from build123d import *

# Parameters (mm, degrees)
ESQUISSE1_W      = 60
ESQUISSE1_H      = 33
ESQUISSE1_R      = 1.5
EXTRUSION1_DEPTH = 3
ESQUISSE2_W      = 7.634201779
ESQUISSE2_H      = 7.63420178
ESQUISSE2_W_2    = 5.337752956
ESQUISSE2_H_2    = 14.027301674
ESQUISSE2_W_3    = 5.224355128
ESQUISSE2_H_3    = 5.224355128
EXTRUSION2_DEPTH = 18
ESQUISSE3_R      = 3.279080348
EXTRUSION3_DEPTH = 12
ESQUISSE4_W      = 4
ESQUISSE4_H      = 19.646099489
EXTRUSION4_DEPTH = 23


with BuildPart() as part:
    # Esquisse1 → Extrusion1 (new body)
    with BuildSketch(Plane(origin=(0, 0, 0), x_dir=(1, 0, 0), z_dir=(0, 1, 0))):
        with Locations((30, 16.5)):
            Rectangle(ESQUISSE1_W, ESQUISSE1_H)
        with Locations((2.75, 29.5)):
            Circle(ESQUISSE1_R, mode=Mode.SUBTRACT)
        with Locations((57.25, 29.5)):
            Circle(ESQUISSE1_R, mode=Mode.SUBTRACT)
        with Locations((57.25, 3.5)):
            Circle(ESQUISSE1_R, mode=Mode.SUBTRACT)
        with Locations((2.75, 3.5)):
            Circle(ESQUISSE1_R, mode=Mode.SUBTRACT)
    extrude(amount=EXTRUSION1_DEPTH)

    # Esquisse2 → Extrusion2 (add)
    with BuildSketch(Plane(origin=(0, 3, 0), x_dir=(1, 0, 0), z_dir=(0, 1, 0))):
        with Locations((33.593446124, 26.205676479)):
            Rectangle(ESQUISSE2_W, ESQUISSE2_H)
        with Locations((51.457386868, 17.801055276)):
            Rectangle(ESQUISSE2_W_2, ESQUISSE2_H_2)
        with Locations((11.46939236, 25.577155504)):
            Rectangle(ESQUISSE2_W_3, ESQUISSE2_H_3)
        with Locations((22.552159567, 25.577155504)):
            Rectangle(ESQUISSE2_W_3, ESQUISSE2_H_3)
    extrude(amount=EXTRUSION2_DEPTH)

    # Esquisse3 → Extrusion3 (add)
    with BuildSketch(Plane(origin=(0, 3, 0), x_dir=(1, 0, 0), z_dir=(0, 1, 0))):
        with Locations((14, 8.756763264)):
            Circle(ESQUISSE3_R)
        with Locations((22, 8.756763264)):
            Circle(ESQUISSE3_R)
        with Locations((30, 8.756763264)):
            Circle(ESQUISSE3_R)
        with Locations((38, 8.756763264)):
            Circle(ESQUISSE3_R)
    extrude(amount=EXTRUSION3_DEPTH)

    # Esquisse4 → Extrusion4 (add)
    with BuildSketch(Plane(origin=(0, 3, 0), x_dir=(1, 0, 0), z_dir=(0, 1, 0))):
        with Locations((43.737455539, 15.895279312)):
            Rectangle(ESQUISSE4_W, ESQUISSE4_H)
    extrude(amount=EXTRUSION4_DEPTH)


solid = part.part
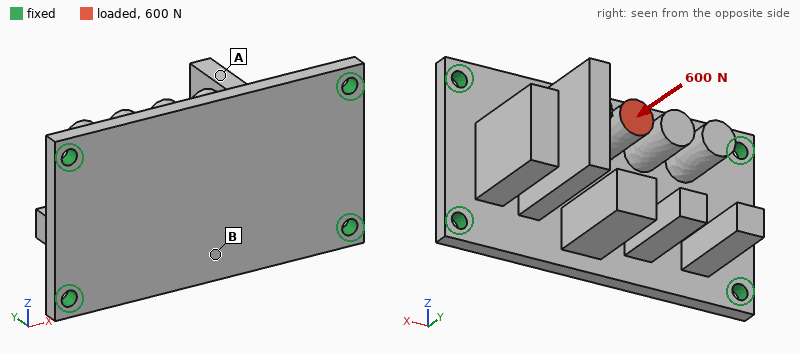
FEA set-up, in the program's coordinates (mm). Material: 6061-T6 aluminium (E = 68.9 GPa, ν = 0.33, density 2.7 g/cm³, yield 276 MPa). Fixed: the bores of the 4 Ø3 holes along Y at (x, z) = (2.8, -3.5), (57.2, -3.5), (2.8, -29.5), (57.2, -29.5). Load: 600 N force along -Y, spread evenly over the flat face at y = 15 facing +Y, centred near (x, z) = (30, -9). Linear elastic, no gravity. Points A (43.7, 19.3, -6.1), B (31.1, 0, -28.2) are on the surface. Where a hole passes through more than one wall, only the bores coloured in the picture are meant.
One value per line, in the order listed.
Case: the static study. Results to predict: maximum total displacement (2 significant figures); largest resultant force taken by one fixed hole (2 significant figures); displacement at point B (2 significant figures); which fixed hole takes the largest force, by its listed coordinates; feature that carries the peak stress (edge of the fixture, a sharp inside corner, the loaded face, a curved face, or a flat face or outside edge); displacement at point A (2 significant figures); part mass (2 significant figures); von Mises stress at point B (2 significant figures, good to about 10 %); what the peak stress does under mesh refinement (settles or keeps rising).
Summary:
0.15 mm
260 N
0.062 mm
(57.2, -3.5)
edge of the fixture
0.12 mm
34 g
32 MPa
keeps rising
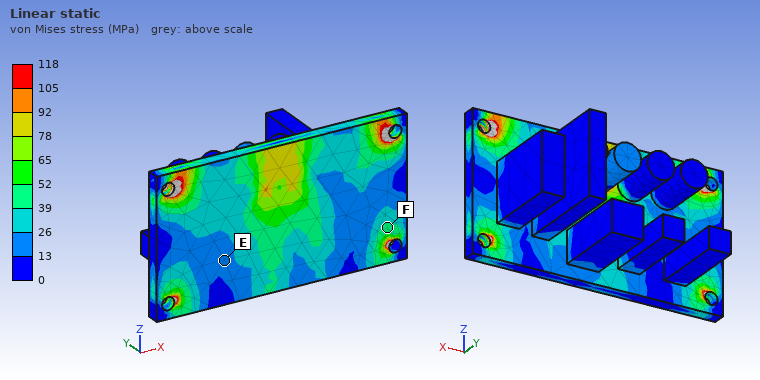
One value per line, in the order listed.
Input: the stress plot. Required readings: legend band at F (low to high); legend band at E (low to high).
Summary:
39 to 52 MPa
13 to 26 MPa
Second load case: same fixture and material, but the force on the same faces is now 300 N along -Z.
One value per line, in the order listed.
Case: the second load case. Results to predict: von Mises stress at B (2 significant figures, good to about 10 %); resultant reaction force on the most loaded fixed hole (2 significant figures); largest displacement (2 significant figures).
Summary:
12 MPa
160 N
0.12 mm
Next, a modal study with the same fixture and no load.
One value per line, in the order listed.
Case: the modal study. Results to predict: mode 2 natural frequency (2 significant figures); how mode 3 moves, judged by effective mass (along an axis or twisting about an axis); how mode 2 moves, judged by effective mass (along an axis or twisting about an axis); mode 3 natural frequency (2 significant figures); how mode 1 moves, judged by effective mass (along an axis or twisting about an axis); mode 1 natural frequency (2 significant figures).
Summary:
4200 Hz
along Y
along Z
5200 Hz
along Y
2800 Hz
